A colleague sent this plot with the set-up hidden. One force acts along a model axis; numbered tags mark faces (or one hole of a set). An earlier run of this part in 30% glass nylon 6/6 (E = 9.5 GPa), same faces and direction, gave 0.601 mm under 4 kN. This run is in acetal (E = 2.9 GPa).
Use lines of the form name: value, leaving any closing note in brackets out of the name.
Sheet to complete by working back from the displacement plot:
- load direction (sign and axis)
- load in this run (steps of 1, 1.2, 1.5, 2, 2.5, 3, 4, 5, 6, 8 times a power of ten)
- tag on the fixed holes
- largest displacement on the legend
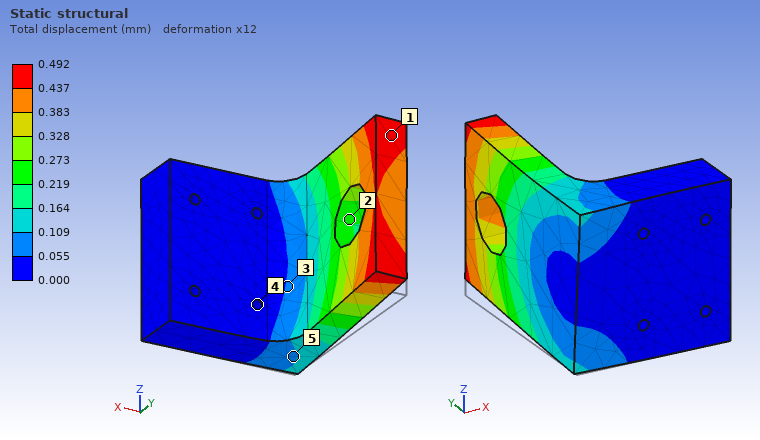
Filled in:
load direction: +Z
load in this run: 1 kN
tag on the fixed holes: 4
largest displacement on the legend: 0.492 mm
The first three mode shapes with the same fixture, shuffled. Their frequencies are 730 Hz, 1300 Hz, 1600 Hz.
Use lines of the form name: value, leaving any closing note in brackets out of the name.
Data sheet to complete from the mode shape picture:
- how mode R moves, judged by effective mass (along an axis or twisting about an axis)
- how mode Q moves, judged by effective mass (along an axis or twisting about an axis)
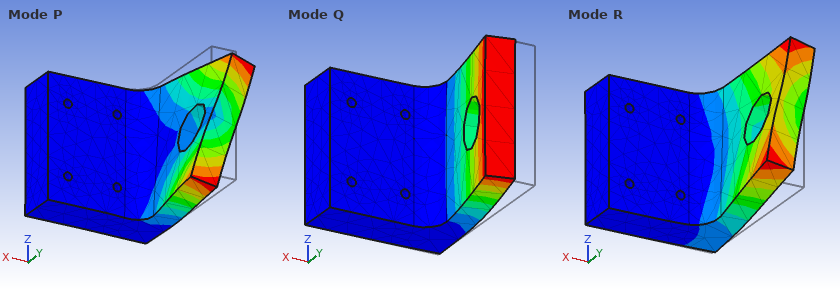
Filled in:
how mode R moves, judged by effective mass: along Z
how mode Q moves, judged by effective mass: along X
